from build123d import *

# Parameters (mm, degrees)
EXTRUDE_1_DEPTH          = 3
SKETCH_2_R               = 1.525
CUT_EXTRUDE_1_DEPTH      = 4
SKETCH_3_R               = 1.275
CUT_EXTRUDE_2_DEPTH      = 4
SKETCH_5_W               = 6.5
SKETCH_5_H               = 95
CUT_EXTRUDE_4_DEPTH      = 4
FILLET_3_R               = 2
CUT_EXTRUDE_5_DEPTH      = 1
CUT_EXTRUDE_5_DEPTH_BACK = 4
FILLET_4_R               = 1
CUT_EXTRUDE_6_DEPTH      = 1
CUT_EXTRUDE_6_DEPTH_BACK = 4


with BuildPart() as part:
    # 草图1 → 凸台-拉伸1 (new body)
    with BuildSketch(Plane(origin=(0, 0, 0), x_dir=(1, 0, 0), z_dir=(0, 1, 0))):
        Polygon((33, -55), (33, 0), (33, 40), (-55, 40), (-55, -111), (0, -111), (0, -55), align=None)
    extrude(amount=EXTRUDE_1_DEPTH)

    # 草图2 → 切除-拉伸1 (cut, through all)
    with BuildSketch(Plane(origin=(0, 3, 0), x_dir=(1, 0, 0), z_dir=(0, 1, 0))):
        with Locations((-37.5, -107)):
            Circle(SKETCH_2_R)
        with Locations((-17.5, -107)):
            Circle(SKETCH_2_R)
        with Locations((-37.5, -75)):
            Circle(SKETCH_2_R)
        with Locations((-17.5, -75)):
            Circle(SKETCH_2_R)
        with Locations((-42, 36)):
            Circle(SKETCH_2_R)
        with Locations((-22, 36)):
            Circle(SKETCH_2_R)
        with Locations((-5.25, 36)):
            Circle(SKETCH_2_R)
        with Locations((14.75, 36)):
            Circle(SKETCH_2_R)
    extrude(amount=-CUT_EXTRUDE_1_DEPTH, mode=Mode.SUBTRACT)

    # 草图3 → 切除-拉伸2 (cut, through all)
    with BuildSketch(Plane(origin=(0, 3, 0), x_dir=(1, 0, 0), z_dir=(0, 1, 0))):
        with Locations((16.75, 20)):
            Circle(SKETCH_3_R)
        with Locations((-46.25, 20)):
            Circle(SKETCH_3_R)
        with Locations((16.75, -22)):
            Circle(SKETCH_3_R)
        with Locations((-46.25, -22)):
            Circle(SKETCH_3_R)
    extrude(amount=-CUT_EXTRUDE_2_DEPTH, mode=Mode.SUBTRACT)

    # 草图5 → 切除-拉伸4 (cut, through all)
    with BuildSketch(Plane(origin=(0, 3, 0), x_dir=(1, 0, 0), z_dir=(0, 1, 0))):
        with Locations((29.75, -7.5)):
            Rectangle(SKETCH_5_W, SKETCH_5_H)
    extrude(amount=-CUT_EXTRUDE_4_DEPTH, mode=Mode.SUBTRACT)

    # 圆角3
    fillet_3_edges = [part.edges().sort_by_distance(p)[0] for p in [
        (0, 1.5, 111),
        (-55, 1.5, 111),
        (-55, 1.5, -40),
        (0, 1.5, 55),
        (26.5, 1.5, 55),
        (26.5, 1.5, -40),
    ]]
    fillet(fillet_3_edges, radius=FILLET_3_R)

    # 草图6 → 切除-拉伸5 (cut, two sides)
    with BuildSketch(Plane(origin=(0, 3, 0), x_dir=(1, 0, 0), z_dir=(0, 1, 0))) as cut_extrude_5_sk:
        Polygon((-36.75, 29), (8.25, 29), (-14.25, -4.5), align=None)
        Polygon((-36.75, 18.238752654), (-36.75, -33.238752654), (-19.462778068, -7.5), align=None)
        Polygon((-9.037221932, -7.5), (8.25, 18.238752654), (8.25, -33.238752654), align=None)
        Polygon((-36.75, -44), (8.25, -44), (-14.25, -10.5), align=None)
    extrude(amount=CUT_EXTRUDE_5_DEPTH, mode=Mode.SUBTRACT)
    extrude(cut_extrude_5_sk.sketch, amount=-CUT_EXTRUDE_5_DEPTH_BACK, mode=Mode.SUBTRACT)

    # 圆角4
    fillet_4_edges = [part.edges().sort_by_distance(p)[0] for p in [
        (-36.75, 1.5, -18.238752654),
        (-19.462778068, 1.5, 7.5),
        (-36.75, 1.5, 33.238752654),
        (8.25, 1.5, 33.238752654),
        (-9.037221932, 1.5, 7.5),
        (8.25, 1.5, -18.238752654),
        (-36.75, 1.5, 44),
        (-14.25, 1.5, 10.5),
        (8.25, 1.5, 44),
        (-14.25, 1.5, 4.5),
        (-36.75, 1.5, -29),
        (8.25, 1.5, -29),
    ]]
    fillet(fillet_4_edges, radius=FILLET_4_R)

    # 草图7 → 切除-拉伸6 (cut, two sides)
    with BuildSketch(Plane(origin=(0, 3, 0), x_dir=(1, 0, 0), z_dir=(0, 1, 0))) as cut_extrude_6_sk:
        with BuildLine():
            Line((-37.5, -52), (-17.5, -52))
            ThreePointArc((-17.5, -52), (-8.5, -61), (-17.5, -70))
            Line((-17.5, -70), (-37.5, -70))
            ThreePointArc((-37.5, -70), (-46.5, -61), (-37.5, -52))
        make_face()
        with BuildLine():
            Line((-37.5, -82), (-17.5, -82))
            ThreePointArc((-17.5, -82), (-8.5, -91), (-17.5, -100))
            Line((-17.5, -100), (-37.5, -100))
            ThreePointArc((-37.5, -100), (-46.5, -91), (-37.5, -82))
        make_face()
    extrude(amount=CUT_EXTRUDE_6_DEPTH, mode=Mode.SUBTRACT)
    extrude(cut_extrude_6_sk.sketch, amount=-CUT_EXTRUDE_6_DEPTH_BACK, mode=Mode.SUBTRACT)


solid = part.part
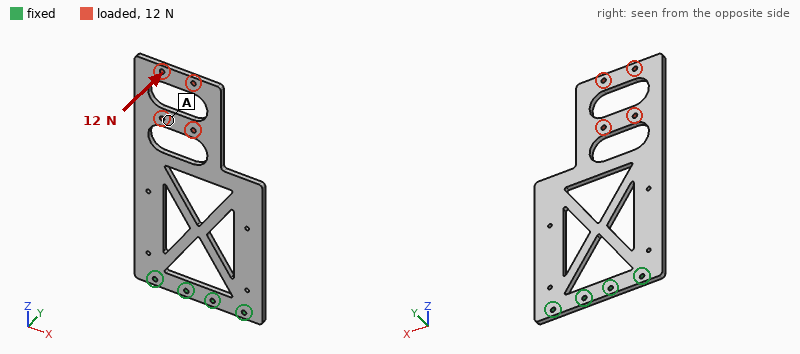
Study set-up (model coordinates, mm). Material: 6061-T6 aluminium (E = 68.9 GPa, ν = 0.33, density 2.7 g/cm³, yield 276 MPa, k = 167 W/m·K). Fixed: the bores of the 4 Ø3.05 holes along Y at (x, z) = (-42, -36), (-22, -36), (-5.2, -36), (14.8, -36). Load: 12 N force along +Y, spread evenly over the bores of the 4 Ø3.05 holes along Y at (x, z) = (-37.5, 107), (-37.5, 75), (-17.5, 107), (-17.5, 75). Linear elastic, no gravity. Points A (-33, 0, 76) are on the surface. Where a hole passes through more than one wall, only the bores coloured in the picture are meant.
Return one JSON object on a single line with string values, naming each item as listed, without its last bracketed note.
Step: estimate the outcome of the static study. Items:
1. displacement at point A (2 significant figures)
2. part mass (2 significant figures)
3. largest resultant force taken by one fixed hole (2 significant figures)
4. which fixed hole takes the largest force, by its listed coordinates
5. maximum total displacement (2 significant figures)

{"displacement at point A": "1.1 mm", "part mass": "58 g", "largest resultant force taken by one fixed hole": "14 N", "which fixed hole takes the largest force, by its listed coordinates": "(-42, -36)", "maximum total displacement": "1.7 mm"}
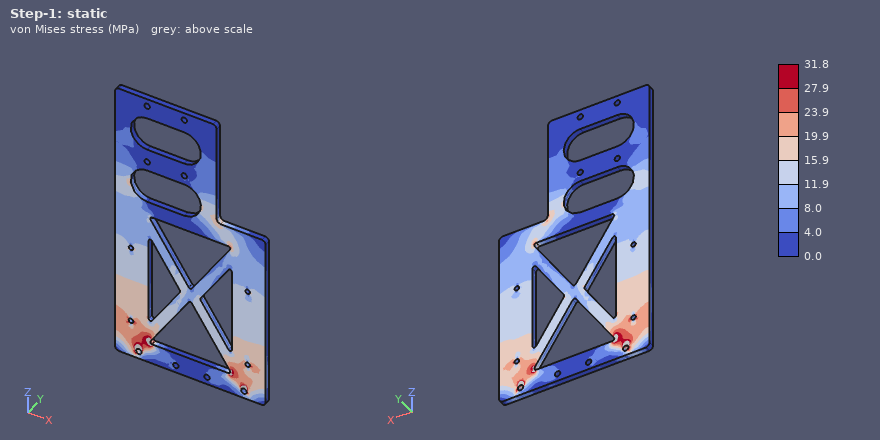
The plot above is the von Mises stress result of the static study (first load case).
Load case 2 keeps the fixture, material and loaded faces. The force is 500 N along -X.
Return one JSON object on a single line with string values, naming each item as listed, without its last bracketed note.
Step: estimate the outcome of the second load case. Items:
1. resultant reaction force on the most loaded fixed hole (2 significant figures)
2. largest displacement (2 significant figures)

{"resultant reaction force on the most loaded fixed hole": "1.1 kN", "largest displacement": "0.20 mm"}
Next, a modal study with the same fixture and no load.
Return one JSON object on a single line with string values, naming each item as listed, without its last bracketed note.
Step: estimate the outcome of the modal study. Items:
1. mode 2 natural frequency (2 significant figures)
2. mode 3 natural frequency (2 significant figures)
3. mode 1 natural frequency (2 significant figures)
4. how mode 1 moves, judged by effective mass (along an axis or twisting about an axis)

{"mode 2 natural frequency": "450 Hz", "mode 3 natural frequency": "580 Hz", "mode 1 natural frequency": "120 Hz", "how mode 1 moves, judged by effective mass": "along Y"}
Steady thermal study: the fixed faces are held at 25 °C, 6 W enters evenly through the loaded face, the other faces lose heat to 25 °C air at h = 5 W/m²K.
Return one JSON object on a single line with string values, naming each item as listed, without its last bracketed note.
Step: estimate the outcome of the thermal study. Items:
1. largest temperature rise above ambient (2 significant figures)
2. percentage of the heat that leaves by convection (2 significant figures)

{"largest temperature rise above ambient": "43 K", "percentage of the heat that leaves by convection": "25 %"}
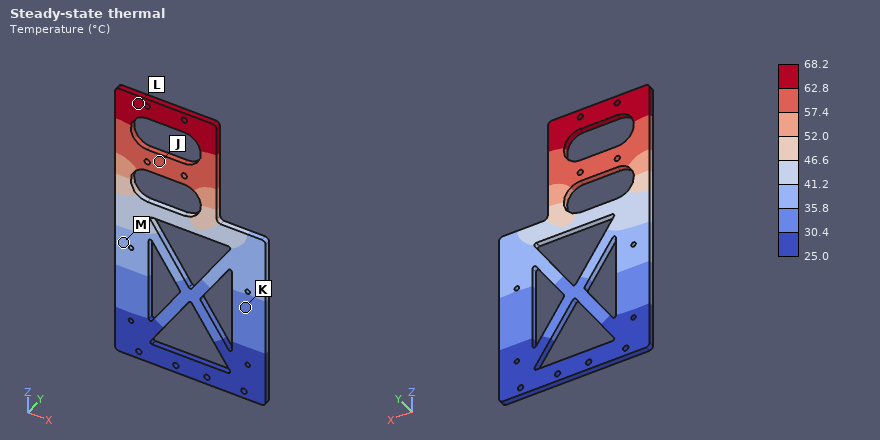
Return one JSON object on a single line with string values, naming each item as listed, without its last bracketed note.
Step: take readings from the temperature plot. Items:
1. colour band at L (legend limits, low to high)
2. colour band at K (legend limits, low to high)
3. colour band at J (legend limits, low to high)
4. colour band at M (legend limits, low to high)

{"colour band at L": "62.8 to 68.2 °C", "colour band at K": "30.4 to 35.8 °C", "colour band at J": "57.4 to 62.8 °C", "colour band at M": "35.8 to 41.2 °C"}
